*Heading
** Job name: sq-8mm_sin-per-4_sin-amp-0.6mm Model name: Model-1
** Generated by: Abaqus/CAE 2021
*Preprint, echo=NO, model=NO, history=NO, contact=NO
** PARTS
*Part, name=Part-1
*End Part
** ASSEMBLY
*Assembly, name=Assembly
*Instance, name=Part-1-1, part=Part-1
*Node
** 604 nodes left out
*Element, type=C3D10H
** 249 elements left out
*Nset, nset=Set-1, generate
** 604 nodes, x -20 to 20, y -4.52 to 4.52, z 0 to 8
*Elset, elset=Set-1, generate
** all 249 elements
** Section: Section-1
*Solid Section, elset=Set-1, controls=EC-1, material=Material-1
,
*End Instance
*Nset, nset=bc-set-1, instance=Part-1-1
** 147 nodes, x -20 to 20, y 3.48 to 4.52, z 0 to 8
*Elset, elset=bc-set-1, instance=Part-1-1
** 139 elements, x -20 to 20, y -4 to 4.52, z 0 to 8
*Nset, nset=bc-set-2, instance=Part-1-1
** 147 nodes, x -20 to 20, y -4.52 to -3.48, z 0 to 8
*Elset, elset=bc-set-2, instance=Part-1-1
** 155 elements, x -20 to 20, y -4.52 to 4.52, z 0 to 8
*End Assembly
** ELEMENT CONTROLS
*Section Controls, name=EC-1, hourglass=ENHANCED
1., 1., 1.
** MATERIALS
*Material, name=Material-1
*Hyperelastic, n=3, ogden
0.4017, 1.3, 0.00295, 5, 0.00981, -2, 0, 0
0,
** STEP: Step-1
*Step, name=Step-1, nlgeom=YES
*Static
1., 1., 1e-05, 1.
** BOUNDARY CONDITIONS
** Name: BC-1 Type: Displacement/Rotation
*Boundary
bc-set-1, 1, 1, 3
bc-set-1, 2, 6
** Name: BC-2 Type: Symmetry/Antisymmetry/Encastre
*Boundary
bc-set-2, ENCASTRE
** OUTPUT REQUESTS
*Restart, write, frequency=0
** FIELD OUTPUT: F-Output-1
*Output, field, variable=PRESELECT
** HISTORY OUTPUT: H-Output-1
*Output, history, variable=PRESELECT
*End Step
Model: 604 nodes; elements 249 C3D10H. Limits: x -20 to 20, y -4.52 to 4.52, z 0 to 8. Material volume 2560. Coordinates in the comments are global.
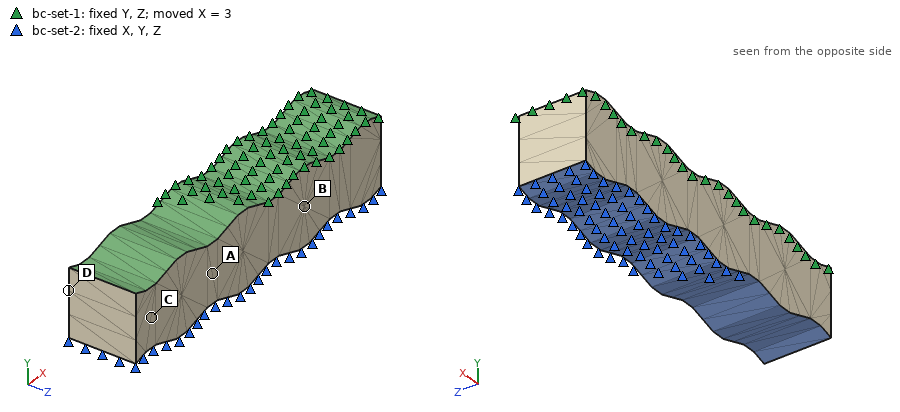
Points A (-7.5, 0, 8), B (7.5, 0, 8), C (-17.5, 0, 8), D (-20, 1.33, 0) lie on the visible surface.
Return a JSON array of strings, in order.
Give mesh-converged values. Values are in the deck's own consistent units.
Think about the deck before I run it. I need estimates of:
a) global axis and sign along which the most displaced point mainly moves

["+X"]
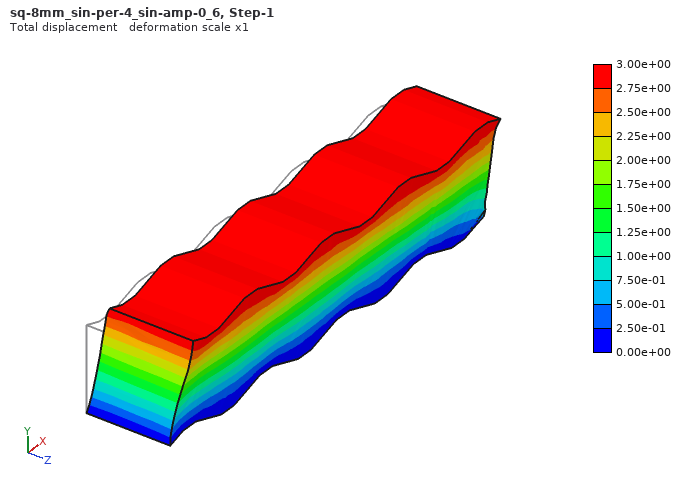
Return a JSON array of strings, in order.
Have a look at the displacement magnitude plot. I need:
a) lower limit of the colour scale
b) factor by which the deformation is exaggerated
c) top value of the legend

["0.00e+00", "1", "3.00e+00"]
